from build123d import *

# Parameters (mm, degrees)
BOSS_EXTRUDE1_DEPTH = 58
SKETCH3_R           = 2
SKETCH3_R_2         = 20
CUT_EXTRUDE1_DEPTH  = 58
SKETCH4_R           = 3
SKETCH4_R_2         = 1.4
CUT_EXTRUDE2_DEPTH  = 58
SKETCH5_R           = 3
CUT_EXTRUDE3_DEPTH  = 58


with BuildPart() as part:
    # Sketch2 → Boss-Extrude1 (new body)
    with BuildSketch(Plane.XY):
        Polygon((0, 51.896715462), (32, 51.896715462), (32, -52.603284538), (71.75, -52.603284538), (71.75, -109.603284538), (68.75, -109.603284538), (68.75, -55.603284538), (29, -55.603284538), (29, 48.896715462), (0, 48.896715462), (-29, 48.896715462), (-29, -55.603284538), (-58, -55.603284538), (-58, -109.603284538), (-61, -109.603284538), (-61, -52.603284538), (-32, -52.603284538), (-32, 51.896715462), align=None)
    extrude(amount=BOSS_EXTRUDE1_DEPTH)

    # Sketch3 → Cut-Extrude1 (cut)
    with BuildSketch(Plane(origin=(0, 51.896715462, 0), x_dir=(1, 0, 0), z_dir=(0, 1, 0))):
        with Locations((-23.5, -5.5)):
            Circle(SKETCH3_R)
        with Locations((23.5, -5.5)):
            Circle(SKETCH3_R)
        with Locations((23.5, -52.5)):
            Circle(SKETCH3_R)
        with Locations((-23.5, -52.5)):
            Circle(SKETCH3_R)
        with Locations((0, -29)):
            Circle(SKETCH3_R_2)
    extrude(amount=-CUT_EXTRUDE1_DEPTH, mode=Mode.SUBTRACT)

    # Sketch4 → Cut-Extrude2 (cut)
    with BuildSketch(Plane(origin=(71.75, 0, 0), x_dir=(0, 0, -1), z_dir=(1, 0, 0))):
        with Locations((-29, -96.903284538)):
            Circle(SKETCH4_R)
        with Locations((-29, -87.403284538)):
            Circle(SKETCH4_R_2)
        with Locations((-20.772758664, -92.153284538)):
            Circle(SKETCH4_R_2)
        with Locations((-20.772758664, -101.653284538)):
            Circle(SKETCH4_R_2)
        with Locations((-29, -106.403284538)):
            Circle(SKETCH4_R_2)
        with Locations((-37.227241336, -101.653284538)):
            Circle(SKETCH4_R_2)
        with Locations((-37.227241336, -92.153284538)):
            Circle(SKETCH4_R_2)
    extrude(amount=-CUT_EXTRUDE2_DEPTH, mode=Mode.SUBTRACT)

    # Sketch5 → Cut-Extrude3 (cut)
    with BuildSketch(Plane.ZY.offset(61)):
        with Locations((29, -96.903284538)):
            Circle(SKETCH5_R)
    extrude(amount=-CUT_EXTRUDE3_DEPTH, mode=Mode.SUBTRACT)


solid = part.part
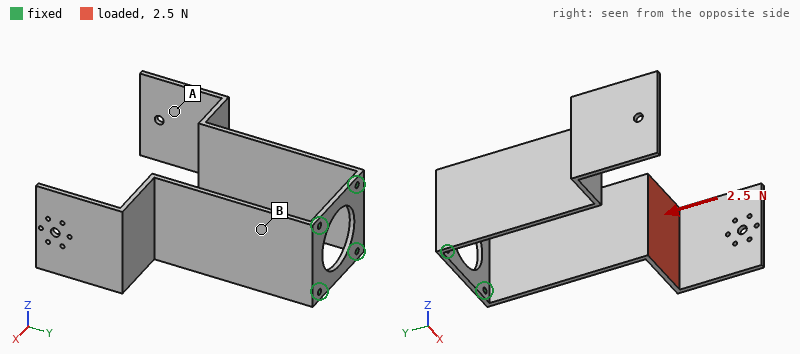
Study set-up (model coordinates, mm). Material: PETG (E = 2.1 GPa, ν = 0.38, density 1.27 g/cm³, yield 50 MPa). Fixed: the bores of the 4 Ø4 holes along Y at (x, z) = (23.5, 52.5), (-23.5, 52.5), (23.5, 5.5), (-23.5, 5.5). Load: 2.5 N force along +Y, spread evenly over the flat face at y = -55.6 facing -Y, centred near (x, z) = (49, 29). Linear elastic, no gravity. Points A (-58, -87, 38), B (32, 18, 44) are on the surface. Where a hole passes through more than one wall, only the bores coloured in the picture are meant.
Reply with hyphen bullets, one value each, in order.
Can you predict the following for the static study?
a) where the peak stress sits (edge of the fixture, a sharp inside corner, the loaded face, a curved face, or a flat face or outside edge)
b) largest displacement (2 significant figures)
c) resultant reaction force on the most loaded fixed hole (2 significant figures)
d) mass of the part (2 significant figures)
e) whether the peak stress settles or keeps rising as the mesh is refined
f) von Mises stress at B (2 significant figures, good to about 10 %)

- edge of the fixture
- 2.3 mm
- 1.3 N
- 94 g
- keeps rising
- 0.52 MPa
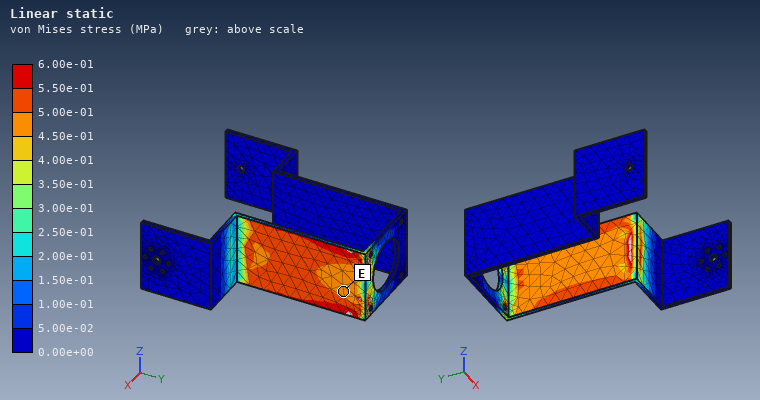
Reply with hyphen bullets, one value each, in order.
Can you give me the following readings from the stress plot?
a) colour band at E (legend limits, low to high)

- 4.50e-01 to 5.00e-01 MPa
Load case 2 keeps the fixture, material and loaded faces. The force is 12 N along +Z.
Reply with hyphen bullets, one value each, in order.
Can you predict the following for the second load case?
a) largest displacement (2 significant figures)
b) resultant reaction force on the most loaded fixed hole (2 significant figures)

- 2.4 mm
- 29 N
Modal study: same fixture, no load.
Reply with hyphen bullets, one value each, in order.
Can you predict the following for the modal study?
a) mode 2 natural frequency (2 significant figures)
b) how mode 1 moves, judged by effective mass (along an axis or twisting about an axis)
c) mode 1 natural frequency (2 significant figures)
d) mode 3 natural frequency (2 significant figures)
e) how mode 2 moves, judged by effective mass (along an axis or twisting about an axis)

- 20 Hz
- along X
- 19 Hz
- 61 Hz
- along X
